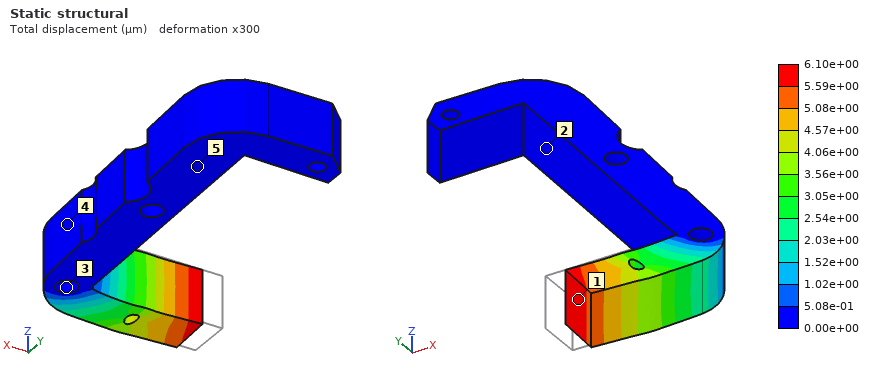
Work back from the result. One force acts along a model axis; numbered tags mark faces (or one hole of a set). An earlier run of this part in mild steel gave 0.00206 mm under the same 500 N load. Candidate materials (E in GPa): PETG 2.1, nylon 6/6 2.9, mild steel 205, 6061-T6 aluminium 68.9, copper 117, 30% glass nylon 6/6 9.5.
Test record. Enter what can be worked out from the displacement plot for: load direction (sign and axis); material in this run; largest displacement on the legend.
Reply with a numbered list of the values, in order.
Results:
1. +X
2. 6061-T6 aluminium
3. 6.10e+00 µm
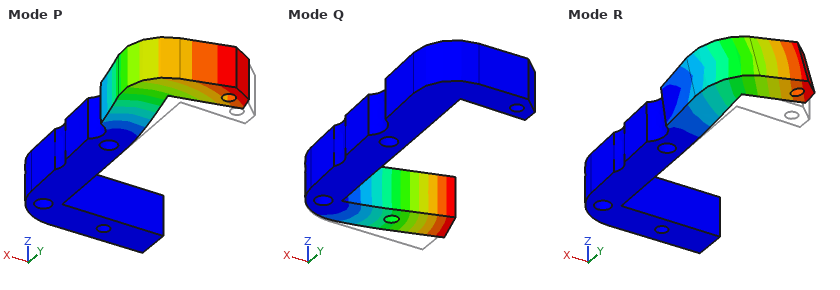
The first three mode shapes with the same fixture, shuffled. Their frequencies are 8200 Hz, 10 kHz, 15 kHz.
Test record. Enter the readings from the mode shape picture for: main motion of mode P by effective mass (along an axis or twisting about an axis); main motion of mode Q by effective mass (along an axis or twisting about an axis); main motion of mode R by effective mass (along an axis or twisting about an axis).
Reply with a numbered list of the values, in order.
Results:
1. along X
2. along Y
3. along Z
